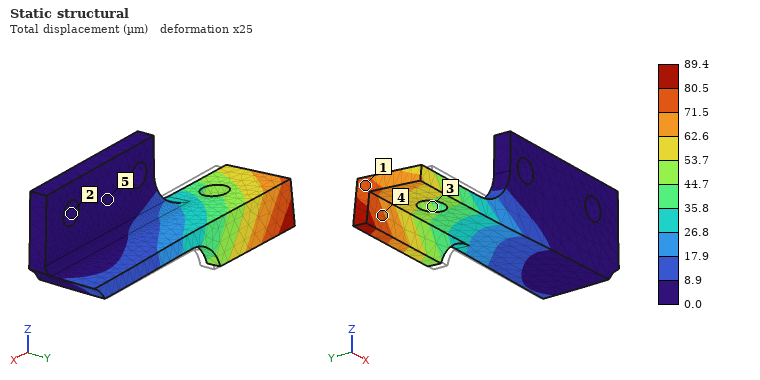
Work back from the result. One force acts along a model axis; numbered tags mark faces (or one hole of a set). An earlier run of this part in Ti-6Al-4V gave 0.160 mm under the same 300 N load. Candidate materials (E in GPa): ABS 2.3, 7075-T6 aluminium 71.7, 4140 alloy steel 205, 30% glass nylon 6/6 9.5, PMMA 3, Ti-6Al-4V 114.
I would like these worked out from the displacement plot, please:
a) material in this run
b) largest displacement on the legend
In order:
4140 alloy steel
89.4 µm
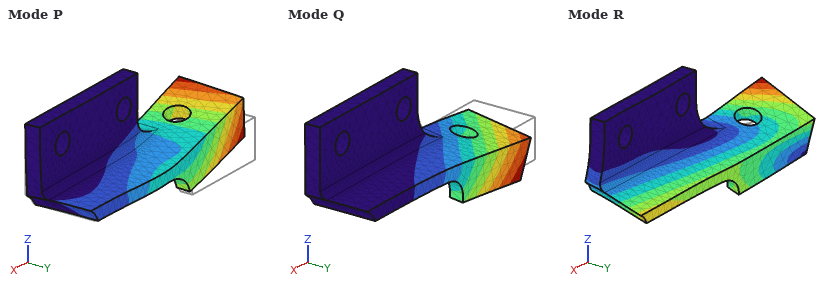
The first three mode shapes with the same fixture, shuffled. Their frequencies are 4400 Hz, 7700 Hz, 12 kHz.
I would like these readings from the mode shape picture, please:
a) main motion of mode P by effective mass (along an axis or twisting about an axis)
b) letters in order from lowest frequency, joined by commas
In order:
along Y
Q, P, R
